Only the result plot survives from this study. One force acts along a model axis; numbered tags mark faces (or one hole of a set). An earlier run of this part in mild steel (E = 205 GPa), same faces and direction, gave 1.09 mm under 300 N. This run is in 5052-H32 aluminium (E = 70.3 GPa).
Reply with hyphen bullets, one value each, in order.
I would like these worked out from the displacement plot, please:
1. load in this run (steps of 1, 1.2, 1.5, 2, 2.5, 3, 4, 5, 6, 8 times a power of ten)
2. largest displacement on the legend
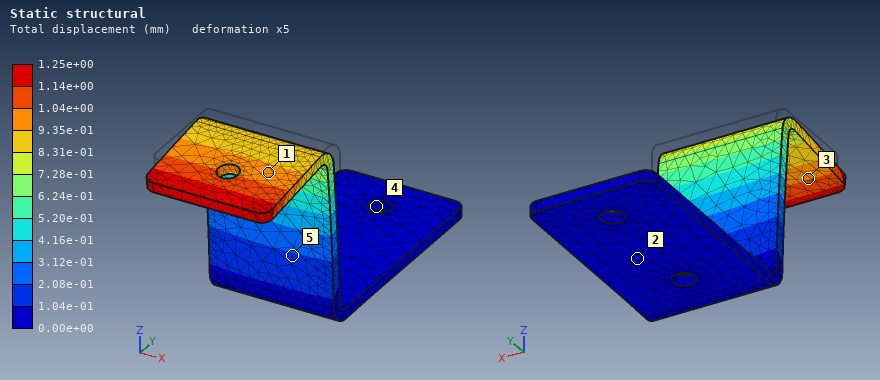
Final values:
- 120 N
- 1.25e+00 mm
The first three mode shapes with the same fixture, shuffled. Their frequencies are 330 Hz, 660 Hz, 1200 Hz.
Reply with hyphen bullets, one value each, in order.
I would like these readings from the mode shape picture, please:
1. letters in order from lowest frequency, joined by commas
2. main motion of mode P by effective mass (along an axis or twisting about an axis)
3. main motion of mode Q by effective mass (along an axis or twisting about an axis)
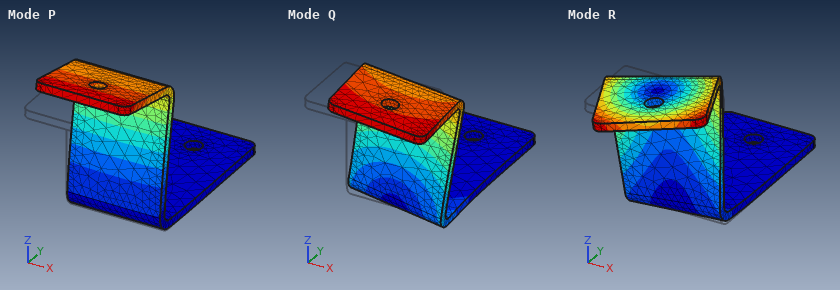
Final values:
- P, Q, R
- along Y
- along X
